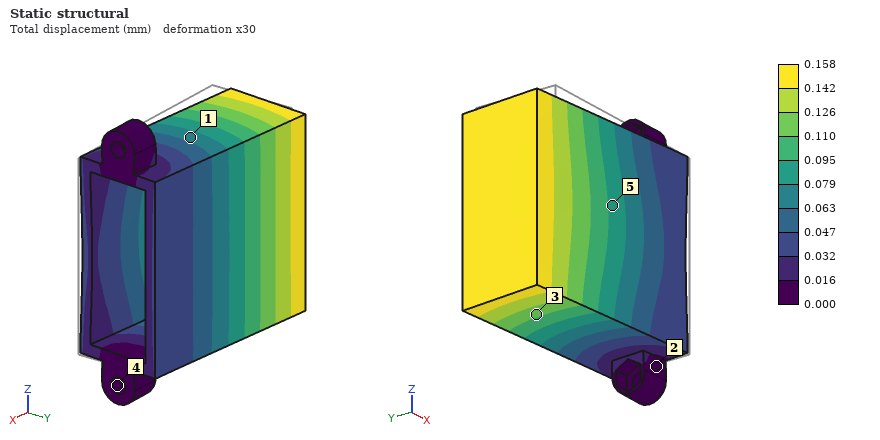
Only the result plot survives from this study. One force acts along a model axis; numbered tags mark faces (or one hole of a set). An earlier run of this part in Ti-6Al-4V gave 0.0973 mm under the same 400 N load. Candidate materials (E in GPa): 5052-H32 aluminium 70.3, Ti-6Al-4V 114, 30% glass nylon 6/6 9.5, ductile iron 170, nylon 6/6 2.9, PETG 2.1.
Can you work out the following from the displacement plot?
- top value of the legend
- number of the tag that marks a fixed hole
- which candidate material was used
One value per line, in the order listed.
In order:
0.158 mm
4
5052-H32 aluminium
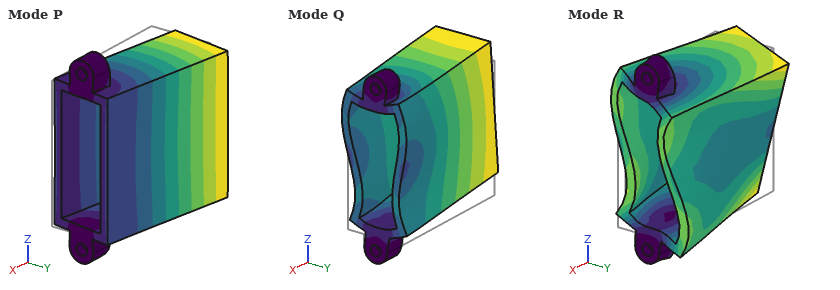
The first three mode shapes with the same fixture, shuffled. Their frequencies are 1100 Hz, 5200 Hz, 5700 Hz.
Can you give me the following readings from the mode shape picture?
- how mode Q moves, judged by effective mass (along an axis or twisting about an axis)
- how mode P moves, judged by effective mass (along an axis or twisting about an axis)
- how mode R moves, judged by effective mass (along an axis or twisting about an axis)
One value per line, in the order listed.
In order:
along Z
along Y
twisting about X
